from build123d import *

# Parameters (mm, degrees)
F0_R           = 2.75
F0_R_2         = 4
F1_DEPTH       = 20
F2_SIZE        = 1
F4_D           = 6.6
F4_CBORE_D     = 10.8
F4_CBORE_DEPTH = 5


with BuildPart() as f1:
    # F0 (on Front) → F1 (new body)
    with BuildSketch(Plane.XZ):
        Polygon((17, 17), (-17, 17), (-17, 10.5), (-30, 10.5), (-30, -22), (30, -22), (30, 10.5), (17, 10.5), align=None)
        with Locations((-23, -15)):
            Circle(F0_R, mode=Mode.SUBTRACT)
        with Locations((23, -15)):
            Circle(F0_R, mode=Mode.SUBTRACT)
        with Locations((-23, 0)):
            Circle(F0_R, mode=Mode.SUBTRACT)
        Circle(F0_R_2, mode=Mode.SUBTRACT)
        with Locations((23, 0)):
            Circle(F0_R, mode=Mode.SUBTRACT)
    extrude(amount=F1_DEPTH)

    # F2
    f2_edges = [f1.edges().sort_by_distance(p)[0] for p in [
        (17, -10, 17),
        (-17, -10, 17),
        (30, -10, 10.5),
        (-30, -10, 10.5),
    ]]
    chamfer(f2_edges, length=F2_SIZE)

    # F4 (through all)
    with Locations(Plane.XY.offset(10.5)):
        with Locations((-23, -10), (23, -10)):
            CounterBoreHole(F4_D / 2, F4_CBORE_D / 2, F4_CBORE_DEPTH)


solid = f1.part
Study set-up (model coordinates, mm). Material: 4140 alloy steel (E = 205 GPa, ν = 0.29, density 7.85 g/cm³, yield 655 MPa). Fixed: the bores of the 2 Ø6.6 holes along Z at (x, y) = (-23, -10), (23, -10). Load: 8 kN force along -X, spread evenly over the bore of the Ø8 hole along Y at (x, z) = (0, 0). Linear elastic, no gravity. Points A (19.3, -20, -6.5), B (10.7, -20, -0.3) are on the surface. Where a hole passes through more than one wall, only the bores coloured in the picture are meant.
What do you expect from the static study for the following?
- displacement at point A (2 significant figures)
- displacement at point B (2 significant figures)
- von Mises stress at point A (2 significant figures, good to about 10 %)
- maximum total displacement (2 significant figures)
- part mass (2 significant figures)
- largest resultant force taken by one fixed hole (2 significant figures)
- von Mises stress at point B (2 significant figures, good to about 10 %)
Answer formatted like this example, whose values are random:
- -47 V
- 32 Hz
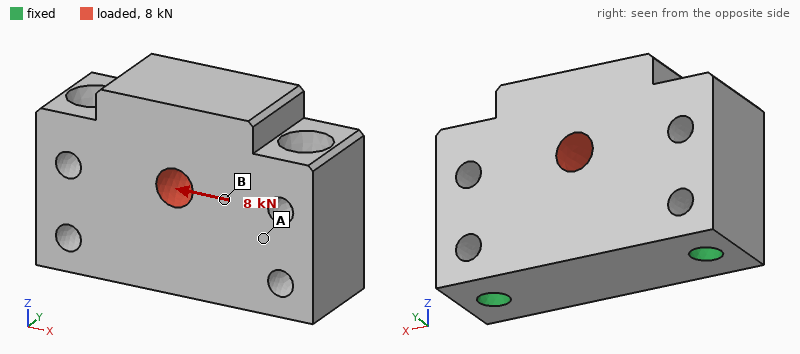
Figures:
- 0.35 µm
- 0.78 µm
- 4.5 MPa
- 1.5 µm
- 300 g
- 4.1 kN
- 12 MPa
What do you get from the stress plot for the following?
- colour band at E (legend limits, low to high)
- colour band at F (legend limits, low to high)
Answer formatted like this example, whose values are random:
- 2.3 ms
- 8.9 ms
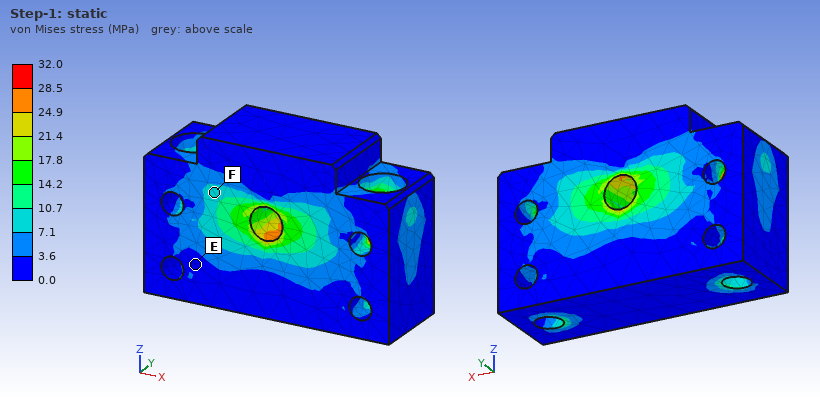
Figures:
- 0.0 to 3.6 MPa
- 7.1 to 10.7 MPa
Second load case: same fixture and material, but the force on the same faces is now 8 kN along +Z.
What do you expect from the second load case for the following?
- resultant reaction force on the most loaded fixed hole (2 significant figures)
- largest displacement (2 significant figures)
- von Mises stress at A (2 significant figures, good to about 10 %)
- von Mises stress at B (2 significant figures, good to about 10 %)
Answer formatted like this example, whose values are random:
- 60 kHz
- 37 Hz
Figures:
- 4.1 kN
- 2.4 µm
- 7.2 MPa
- 10 MPa
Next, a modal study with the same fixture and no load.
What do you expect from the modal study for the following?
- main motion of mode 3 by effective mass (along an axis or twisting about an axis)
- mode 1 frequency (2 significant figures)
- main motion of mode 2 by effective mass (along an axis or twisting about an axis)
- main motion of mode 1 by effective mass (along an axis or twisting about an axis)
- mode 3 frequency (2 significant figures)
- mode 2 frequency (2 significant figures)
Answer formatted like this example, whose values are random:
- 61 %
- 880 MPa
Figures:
- along Z
- 17 kHz
- along Y
- along Y
- 28 kHz
- 26 kHz
